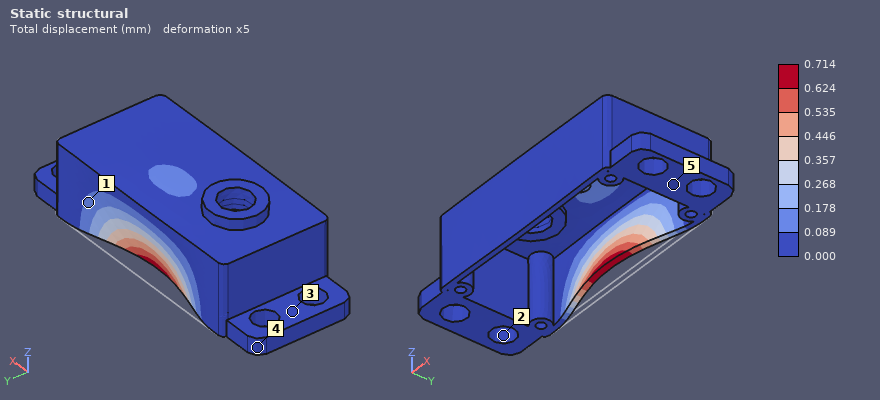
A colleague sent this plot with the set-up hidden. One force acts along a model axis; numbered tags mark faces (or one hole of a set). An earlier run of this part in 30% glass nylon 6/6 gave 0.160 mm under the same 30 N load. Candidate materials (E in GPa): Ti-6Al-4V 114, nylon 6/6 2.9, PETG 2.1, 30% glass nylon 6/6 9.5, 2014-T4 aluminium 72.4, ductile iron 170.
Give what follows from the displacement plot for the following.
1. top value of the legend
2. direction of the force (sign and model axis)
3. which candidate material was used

0.714 mm
-Y
PETG
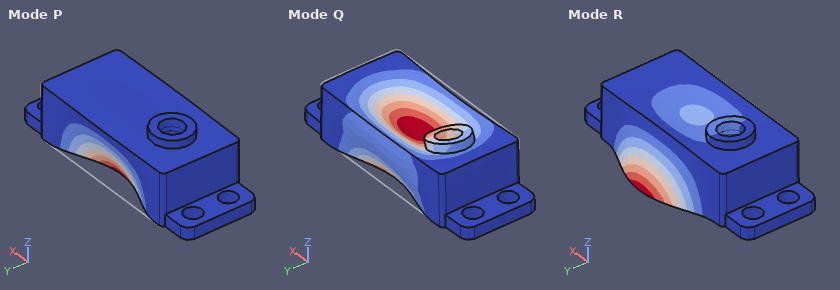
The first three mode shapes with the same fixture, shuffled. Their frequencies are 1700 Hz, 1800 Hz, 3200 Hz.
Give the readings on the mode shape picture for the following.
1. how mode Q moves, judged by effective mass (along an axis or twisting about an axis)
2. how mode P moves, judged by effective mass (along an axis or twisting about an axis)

along Z
along Y
